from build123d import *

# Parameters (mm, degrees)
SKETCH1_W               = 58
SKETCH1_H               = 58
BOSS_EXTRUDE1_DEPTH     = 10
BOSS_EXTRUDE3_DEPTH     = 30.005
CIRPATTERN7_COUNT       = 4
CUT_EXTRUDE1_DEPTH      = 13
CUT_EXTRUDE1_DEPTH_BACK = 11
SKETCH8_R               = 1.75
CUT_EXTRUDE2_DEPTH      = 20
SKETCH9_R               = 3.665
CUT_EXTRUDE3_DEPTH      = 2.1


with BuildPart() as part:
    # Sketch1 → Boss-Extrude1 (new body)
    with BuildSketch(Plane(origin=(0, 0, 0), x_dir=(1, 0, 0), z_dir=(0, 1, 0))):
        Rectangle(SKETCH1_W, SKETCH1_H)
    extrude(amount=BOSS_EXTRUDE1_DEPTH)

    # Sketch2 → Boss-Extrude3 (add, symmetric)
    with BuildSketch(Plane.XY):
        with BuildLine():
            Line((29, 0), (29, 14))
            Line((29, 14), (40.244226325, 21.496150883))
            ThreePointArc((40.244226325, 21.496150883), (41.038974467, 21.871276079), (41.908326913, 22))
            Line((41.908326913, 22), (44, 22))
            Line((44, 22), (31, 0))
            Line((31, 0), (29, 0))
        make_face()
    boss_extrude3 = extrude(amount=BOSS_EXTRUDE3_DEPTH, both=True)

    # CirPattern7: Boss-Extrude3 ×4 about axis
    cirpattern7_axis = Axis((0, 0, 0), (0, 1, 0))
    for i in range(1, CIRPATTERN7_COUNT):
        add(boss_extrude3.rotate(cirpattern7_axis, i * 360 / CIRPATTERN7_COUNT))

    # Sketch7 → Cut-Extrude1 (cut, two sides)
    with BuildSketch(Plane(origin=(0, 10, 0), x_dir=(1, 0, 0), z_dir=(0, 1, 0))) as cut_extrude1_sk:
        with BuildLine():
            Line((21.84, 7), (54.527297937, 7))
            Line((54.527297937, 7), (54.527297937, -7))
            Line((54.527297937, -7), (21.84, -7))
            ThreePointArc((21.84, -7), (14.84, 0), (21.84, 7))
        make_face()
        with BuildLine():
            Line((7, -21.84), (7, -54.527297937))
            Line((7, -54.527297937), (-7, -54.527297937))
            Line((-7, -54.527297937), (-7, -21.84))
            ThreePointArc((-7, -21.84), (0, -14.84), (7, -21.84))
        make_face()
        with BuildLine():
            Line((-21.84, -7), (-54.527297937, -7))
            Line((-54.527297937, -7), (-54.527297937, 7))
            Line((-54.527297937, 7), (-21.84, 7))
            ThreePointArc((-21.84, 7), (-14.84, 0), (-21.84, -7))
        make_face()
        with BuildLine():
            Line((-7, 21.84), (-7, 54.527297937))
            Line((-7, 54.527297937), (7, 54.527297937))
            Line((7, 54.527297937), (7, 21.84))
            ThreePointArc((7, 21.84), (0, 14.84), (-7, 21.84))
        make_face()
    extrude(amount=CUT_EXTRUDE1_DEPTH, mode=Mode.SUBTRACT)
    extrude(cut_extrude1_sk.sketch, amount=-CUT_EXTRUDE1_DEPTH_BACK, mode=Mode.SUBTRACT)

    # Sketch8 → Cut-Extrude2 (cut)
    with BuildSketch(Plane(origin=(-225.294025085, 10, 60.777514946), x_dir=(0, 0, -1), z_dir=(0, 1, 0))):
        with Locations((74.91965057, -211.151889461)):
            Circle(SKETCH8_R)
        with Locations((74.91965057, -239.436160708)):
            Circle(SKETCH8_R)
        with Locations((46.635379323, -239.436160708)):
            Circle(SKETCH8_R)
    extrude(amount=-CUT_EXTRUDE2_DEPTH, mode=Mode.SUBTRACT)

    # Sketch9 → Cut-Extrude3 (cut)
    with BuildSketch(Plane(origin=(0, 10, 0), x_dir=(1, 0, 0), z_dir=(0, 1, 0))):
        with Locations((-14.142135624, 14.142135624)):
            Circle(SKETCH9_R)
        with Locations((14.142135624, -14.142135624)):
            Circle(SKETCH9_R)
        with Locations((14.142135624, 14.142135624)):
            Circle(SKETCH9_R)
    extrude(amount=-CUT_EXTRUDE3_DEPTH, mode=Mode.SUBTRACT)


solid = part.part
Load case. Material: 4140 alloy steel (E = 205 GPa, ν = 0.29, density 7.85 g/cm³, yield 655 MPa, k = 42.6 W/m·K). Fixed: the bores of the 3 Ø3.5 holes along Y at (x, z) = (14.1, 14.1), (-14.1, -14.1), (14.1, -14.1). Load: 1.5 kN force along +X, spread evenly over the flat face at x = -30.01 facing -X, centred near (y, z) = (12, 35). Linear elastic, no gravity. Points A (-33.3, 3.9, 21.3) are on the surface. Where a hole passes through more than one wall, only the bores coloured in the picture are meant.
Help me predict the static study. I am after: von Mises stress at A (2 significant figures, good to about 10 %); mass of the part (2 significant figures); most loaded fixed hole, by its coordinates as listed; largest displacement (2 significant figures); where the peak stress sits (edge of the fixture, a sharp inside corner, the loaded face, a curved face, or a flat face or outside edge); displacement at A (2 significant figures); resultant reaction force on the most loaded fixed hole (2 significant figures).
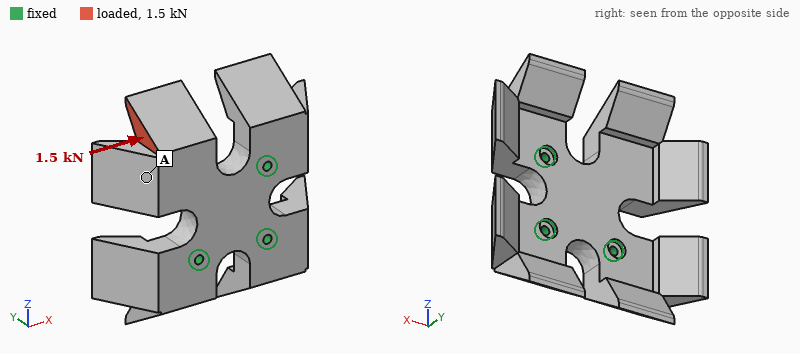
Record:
12 MPa
400 g
(14.1, 14.1)
56 µm
a curved face
32 µm
1.6 kN
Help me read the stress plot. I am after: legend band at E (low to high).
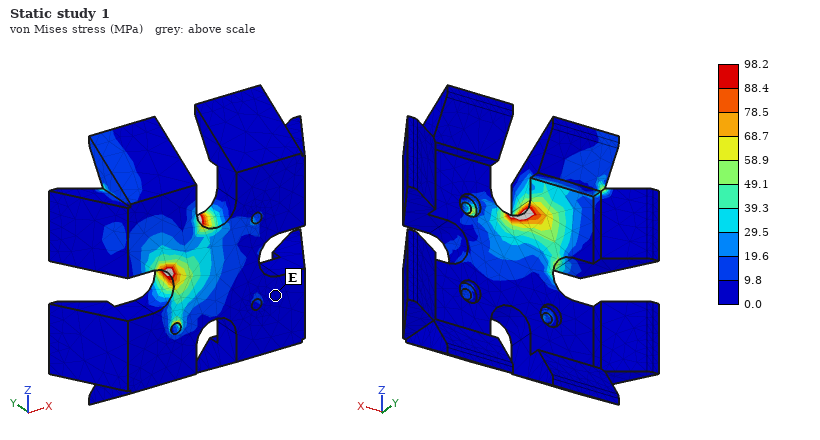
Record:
0.0 to 9.8 MPa
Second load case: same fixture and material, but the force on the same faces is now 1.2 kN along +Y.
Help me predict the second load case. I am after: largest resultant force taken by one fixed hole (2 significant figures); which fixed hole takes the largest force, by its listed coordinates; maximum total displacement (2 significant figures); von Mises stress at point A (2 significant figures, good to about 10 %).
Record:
1.4 kN
(14.1, 14.1)
0.19 mm
22 MPa
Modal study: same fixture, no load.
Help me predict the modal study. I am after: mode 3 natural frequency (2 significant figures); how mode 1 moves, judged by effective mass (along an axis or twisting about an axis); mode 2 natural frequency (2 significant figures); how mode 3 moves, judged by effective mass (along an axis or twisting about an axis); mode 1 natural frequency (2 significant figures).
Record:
5600 Hz
along Y
4400 Hz
along Y
2300 Hz
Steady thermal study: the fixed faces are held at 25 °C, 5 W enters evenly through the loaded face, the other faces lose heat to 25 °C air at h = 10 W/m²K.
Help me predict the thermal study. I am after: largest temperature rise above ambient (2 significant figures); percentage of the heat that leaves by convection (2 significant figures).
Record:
30 K
16 %
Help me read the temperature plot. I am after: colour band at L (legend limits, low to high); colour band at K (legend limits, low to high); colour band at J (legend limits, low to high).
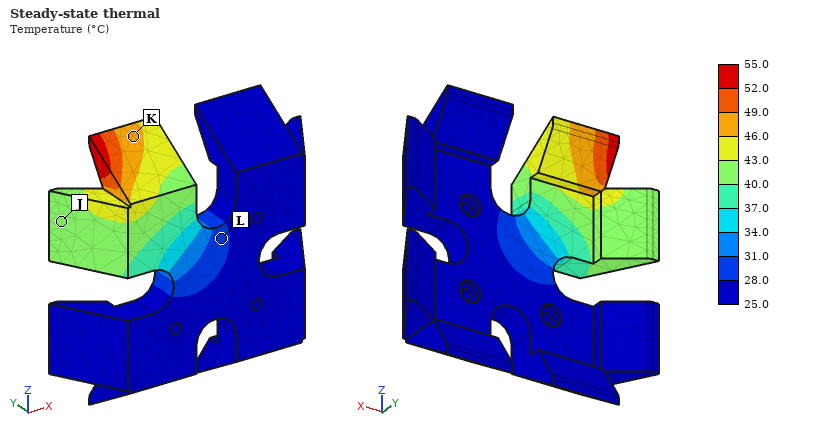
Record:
28.0 to 31.0 °C
46.0 to 49.0 °C
40.0 to 43.0 °C
